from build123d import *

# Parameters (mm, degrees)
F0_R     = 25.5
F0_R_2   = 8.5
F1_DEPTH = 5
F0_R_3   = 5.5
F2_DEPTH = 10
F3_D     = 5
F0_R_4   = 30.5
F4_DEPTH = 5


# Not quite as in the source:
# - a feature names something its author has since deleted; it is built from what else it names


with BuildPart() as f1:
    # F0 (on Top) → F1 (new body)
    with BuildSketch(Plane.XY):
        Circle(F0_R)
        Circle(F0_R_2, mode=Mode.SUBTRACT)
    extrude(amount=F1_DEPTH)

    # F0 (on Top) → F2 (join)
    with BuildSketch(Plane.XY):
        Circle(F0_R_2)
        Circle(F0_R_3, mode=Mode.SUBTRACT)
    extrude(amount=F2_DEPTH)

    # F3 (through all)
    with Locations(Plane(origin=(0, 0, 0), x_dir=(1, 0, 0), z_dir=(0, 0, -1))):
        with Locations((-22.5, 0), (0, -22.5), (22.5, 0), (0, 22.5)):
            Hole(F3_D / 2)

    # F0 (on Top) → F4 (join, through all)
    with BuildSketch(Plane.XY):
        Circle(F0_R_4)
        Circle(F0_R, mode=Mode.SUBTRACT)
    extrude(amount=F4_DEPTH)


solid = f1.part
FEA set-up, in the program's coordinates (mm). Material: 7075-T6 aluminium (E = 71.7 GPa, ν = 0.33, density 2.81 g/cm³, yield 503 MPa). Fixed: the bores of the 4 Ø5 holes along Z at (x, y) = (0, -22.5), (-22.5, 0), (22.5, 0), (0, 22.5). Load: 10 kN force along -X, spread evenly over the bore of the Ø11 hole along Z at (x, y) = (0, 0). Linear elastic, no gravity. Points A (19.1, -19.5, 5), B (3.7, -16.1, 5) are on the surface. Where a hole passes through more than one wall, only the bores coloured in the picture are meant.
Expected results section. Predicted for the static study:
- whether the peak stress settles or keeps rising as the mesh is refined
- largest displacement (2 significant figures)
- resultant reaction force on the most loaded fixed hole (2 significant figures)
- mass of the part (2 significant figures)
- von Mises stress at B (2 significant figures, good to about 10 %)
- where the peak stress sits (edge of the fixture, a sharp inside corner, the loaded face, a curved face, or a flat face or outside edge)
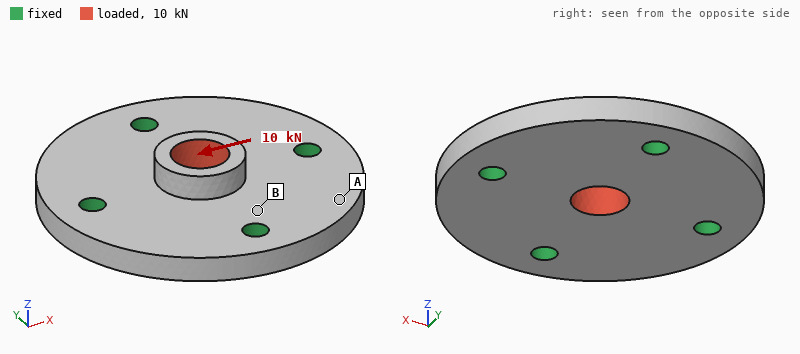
keeps rising
32 µm
3.3 kN
40 g
25 MPa
edge of the fixture
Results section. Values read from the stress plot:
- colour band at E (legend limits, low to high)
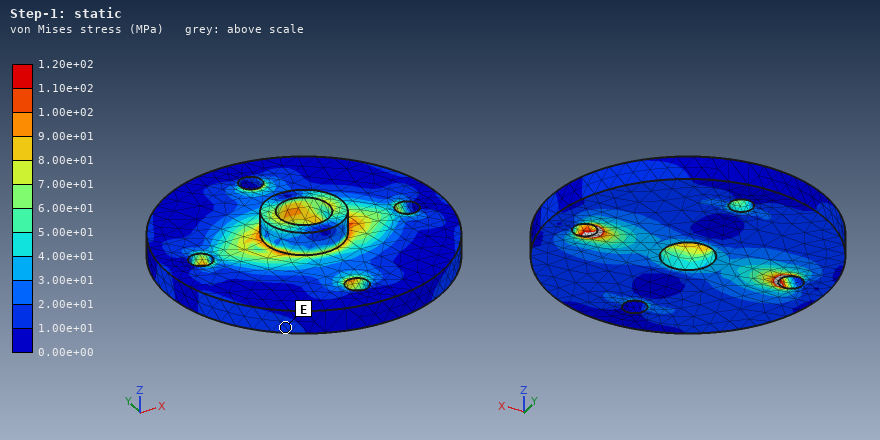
1.00e+01 to 2.00e+01 MPa
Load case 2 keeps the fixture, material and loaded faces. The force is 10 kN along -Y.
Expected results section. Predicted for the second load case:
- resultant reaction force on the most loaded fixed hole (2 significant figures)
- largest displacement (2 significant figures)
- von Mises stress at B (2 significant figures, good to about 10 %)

3.3 kN
32 µm
47 MPa
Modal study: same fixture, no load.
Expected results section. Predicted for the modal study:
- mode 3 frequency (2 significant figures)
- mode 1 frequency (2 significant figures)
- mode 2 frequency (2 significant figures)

17 kHz
16 kHz
17 kHz
